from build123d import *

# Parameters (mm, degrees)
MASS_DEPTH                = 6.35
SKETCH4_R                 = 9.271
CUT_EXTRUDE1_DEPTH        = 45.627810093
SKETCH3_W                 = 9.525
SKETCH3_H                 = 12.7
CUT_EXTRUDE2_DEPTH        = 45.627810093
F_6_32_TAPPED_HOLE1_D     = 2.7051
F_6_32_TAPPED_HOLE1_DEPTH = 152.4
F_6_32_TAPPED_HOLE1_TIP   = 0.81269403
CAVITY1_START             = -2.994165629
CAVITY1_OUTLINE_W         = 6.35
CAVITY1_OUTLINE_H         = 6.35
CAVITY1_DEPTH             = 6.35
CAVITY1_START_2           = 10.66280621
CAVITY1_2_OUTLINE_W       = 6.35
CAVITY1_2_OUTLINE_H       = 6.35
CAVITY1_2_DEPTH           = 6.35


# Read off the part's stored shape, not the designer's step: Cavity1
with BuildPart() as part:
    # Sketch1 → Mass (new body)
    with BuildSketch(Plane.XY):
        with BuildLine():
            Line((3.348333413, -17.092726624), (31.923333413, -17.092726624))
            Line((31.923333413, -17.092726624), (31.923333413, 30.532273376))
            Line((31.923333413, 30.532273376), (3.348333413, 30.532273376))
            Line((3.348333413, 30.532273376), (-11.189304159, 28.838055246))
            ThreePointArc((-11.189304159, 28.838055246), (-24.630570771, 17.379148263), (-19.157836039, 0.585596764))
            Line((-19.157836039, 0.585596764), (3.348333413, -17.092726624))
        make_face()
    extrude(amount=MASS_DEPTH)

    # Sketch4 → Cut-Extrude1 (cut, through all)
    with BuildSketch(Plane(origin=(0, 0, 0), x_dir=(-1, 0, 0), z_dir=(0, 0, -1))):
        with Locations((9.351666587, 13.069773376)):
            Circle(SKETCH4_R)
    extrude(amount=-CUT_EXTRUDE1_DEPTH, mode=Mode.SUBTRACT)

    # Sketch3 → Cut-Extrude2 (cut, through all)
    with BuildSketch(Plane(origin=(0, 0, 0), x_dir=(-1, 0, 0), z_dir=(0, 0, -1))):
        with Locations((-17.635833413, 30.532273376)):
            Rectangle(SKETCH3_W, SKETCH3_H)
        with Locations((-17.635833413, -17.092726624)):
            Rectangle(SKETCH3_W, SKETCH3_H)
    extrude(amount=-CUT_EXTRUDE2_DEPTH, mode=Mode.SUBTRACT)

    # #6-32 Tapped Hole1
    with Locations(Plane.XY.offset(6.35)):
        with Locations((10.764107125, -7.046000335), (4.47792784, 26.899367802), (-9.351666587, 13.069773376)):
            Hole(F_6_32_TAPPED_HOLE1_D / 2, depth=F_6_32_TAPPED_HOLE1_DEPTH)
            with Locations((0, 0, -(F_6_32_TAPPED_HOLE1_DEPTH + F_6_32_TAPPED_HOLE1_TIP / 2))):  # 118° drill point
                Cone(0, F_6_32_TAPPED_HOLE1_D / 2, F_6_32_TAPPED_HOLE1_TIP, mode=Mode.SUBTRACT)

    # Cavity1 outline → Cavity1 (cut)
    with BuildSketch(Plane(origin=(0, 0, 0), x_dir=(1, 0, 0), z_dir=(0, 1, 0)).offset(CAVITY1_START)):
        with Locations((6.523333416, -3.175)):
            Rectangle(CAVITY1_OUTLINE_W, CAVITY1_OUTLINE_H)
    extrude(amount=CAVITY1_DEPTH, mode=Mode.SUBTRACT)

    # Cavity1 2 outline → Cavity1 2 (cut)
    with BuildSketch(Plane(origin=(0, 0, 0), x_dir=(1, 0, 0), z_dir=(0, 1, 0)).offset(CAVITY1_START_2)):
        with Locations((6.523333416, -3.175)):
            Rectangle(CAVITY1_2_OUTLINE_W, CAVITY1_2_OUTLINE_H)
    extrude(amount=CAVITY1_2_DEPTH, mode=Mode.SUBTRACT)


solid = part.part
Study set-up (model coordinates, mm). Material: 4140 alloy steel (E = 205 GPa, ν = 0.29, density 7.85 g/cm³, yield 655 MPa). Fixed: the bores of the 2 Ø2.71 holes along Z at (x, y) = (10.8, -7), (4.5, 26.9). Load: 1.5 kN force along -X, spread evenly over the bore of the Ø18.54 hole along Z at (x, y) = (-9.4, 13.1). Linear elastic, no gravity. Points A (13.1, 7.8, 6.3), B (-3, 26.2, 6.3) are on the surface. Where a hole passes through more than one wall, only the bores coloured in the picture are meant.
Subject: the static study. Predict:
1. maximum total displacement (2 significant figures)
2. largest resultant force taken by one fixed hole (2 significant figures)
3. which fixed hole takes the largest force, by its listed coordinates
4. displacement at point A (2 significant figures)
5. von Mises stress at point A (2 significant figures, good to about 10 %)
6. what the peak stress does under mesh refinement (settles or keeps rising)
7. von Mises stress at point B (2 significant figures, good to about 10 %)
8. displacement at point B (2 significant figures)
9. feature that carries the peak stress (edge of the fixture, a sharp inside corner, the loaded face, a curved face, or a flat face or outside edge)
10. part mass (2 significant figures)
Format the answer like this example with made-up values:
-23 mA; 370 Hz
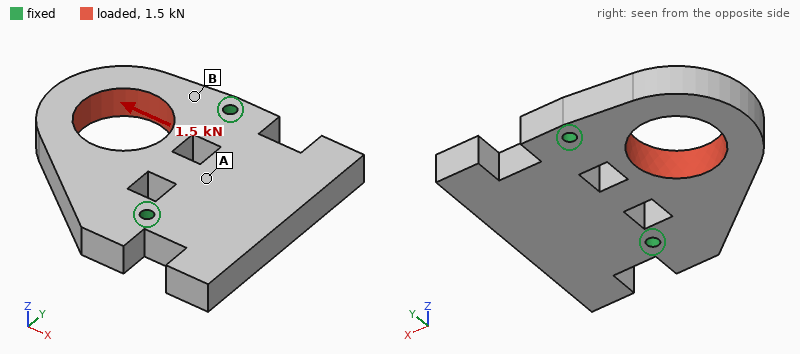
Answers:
2.1 µm; 890 N; (4.5, 26.9); 0.62 µm; 4.8 MPa; keeps rising; 13 MPa; 0.49 µm; edge of the fixture; 91 g
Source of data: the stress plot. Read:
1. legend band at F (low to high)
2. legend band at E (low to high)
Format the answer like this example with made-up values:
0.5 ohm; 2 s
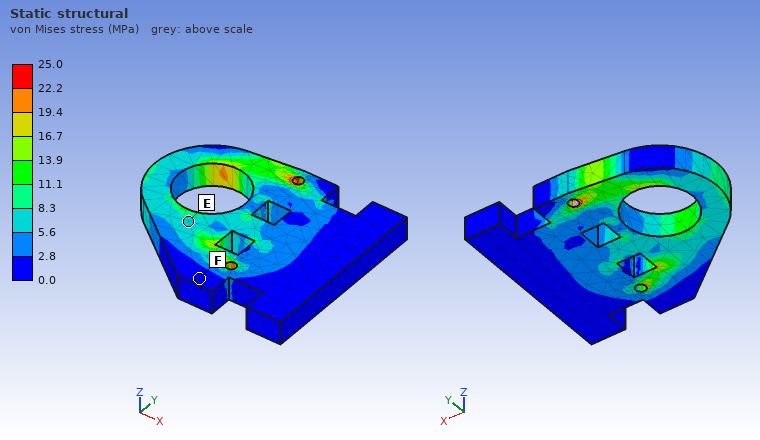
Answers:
0.0 to 2.8 MPa; 5.6 to 8.3 MPa
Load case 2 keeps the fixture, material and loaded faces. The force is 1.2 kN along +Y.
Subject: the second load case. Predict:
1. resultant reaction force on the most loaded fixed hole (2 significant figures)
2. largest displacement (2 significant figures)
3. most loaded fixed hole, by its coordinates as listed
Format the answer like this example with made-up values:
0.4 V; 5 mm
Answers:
930 N; 5.7 µm; (4.5, 26.9)
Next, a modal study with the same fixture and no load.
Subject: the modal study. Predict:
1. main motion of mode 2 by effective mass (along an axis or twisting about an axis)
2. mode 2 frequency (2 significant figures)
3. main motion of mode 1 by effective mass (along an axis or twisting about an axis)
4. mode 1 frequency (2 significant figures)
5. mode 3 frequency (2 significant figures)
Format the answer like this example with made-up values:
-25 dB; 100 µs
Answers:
along Z; 6300 Hz; twisting about Y; 4800 Hz; 11 kHz
